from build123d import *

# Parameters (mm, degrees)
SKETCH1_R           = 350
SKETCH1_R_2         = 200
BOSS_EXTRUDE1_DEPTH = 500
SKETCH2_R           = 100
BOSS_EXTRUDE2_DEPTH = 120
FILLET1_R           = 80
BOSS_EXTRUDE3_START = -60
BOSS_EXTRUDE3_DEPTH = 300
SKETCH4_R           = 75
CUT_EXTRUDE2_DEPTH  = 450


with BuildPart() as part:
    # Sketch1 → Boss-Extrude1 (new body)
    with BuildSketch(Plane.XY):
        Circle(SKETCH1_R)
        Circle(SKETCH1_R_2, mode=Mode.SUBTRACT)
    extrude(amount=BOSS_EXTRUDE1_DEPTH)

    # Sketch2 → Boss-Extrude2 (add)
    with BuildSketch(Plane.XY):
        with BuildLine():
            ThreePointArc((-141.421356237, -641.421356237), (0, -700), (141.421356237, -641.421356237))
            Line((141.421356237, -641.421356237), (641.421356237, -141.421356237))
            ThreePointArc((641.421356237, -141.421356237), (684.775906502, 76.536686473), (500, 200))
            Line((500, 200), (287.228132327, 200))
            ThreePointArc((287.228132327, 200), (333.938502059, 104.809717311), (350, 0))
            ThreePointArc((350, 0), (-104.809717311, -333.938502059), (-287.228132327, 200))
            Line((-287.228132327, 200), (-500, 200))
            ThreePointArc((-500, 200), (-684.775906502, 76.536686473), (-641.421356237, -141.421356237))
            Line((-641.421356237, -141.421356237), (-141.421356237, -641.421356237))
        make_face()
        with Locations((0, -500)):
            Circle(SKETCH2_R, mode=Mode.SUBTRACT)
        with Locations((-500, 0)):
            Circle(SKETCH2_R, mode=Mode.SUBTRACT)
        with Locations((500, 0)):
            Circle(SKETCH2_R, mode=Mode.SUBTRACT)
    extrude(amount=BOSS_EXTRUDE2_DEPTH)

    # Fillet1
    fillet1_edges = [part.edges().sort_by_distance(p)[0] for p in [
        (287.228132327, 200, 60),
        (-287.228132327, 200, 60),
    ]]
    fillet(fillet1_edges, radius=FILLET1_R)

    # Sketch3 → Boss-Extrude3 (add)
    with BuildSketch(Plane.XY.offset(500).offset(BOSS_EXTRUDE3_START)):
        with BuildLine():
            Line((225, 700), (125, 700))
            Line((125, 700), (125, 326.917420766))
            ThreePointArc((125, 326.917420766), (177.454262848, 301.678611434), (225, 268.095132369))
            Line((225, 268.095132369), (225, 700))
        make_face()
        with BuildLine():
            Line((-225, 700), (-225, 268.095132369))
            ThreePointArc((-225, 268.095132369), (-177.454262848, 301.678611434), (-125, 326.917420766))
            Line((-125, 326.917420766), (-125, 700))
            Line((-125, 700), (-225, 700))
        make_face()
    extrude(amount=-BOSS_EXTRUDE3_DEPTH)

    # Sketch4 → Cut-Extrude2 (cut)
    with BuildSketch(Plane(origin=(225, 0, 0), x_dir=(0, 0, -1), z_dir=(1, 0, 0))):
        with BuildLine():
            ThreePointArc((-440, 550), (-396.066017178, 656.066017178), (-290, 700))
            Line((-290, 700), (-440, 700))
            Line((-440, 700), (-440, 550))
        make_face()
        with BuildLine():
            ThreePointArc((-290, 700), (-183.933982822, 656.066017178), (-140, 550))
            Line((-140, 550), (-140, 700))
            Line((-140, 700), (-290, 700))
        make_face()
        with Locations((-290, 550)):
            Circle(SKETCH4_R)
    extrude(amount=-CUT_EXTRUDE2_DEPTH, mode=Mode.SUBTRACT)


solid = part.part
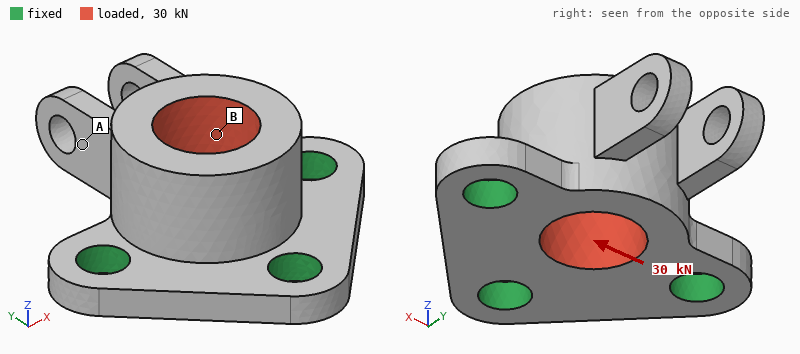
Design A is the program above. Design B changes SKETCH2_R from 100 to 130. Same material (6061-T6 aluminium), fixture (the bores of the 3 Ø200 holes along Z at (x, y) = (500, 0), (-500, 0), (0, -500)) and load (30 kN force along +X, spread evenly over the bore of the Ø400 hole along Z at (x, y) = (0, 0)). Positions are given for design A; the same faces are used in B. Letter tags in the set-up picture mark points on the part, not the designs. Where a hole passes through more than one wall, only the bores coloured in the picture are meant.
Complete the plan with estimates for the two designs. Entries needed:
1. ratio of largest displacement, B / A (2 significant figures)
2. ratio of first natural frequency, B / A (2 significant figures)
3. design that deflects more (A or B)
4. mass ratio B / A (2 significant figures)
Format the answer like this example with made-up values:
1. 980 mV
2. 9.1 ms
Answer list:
1. 0.83
2. 1.1
3. A
4. 0.96
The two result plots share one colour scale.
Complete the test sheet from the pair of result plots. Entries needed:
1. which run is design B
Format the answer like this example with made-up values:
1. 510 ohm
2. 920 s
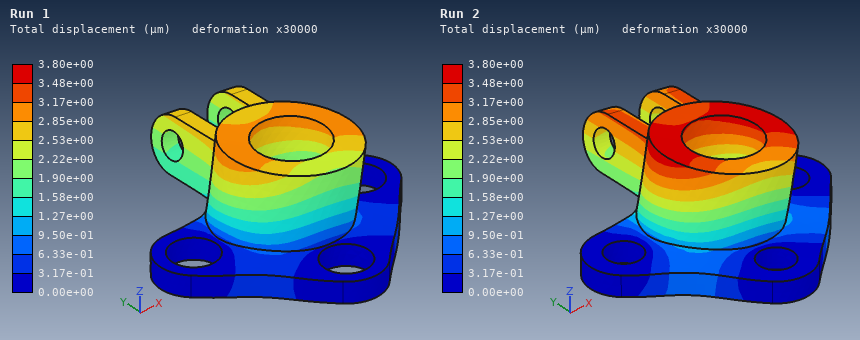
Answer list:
1. Run 1
